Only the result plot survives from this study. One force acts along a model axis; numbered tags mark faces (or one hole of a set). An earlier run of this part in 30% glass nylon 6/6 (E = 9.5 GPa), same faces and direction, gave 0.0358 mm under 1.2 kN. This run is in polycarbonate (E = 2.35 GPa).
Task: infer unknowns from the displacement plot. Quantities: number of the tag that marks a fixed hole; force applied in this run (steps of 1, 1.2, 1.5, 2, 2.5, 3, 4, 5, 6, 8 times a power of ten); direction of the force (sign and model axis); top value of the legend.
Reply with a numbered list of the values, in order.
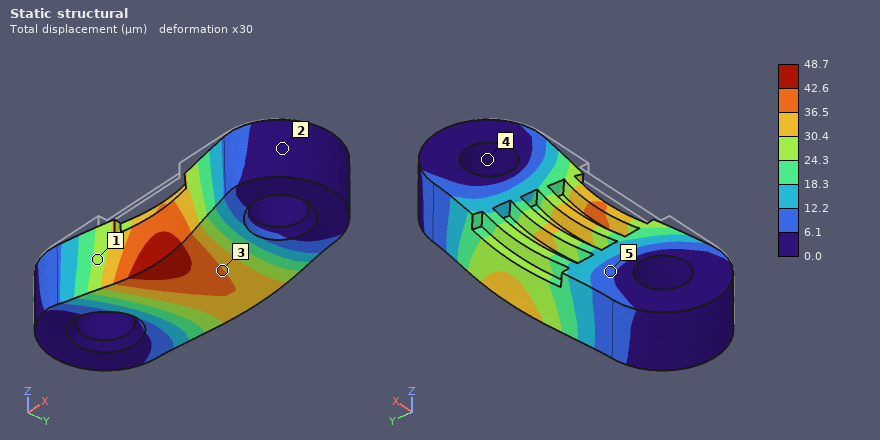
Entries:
1. 4
2. 400 N
3. +Y
4. 48.7 µm
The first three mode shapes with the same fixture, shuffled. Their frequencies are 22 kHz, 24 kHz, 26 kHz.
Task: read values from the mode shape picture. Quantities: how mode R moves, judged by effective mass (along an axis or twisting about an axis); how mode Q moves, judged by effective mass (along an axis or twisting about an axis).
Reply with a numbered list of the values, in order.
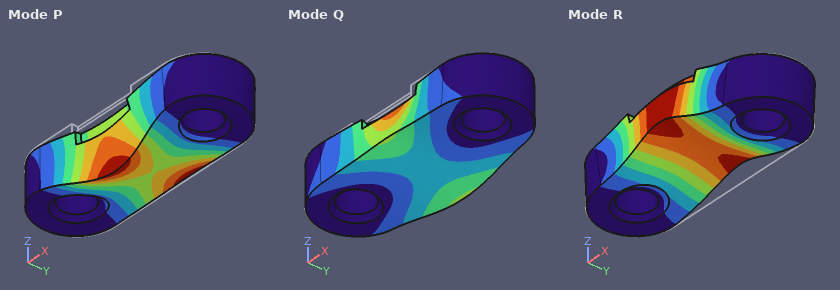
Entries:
1. along Z
2. along Y
